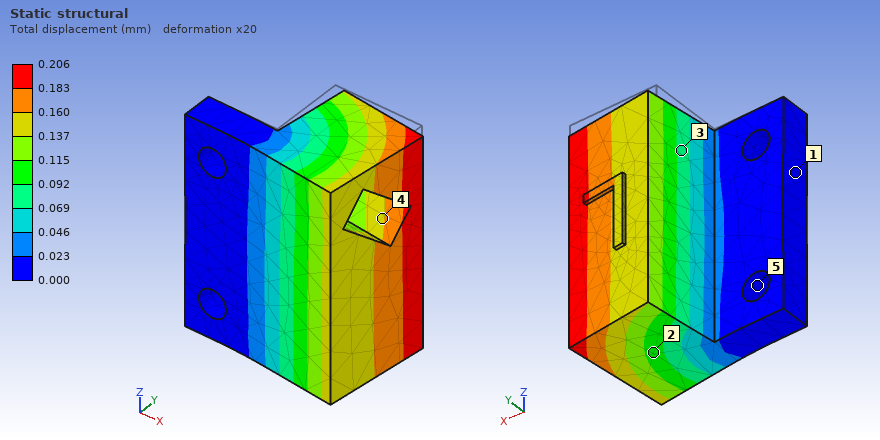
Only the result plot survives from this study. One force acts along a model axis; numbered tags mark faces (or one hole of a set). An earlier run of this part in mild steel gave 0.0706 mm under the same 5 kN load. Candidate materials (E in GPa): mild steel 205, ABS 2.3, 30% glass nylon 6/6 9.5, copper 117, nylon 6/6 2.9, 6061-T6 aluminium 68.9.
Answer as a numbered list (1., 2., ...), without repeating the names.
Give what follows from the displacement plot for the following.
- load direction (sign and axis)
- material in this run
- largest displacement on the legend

1. +X
2. 6061-T6 aluminium
3. 0.206 mm
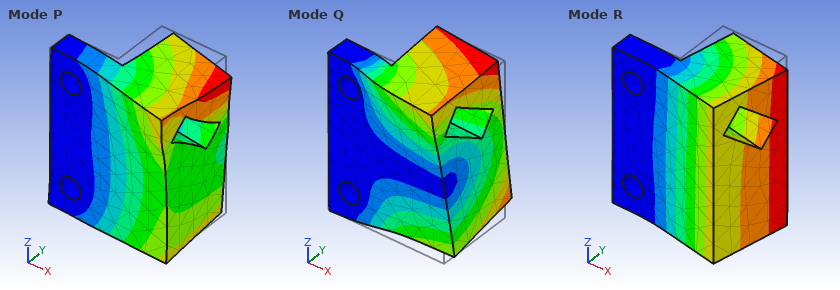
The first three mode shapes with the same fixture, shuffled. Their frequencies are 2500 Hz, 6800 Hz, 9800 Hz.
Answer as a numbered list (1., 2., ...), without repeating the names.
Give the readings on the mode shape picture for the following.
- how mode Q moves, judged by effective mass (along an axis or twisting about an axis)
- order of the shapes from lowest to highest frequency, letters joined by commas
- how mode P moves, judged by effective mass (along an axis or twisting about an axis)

1. along Z
2. R, Q, P
3. along Z
